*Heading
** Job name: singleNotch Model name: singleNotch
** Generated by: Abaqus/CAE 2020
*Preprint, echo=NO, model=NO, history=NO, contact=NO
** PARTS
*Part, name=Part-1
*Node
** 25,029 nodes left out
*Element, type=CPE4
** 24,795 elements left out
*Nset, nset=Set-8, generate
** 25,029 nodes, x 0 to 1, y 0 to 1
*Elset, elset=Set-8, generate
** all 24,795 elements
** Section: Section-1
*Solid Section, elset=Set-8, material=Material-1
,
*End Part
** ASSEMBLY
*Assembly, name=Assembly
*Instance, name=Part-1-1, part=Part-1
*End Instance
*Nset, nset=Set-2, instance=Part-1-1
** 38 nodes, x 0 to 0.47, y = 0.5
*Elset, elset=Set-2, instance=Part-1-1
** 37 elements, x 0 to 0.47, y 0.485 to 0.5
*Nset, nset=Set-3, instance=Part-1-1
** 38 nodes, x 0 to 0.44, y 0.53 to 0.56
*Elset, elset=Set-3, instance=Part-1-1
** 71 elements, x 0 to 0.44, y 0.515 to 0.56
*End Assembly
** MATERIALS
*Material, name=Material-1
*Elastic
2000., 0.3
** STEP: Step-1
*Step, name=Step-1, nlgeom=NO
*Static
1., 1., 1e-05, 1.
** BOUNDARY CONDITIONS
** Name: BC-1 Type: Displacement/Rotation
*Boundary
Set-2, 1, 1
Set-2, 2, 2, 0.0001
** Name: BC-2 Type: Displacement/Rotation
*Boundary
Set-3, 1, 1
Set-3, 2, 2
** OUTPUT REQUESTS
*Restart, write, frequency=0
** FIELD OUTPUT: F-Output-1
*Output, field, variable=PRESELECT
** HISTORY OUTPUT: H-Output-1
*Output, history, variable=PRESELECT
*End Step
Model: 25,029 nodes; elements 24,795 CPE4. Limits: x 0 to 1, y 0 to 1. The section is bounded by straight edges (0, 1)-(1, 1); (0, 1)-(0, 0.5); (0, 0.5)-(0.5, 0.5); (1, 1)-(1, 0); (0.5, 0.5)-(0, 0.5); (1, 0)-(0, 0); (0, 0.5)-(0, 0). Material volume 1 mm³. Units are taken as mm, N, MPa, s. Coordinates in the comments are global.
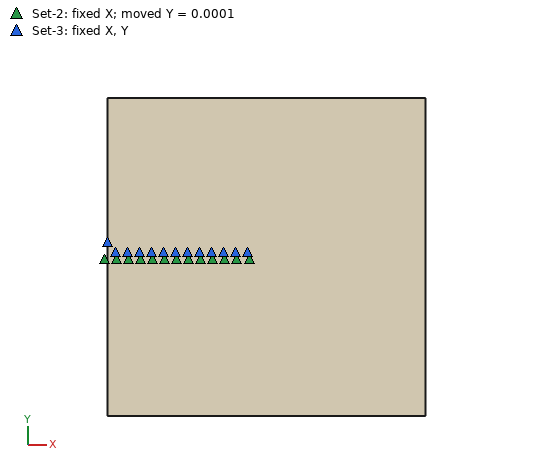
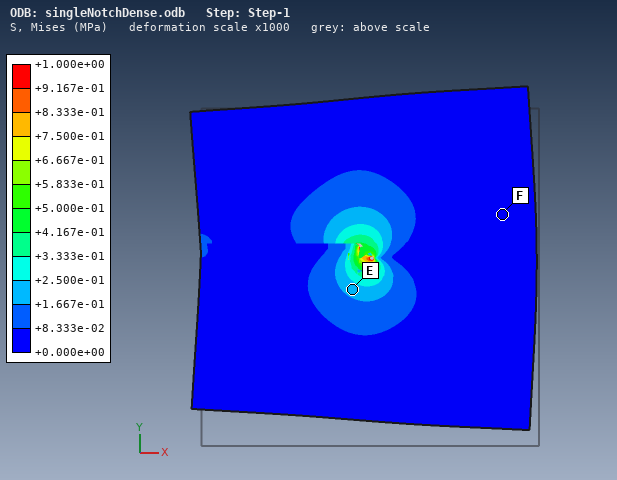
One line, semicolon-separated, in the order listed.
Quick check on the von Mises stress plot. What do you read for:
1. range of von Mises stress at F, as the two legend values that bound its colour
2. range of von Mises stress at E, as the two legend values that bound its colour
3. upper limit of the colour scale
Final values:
+0.000e+00 to +8.333e-02 MPa; +1.667e-01 to +2.500e-01 MPa; +1.000e+00 MPa
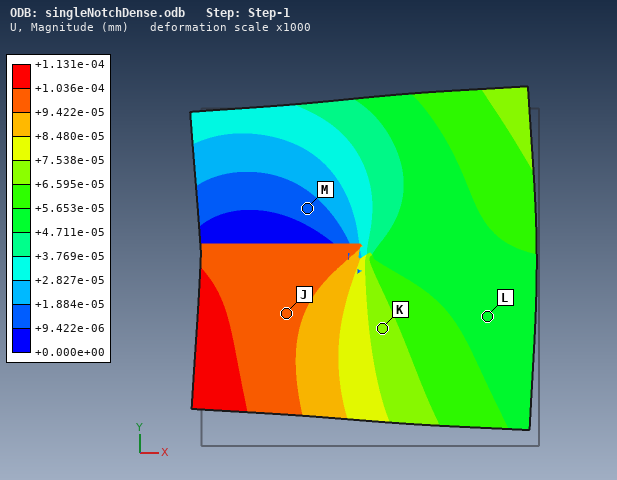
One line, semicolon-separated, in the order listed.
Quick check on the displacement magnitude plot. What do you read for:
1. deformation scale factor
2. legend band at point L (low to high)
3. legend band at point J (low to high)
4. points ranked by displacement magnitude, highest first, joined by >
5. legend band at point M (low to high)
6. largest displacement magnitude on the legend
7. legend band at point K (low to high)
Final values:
1000; +4.711e-05 to +5.653e-05 mm; +9.422e-05 to +1.036e-04 mm; J > K > L > M; +9.422e-06 to +1.884e-05 mm; +1.131e-04 mm; +6.595e-05 to +7.538e-05 mm
